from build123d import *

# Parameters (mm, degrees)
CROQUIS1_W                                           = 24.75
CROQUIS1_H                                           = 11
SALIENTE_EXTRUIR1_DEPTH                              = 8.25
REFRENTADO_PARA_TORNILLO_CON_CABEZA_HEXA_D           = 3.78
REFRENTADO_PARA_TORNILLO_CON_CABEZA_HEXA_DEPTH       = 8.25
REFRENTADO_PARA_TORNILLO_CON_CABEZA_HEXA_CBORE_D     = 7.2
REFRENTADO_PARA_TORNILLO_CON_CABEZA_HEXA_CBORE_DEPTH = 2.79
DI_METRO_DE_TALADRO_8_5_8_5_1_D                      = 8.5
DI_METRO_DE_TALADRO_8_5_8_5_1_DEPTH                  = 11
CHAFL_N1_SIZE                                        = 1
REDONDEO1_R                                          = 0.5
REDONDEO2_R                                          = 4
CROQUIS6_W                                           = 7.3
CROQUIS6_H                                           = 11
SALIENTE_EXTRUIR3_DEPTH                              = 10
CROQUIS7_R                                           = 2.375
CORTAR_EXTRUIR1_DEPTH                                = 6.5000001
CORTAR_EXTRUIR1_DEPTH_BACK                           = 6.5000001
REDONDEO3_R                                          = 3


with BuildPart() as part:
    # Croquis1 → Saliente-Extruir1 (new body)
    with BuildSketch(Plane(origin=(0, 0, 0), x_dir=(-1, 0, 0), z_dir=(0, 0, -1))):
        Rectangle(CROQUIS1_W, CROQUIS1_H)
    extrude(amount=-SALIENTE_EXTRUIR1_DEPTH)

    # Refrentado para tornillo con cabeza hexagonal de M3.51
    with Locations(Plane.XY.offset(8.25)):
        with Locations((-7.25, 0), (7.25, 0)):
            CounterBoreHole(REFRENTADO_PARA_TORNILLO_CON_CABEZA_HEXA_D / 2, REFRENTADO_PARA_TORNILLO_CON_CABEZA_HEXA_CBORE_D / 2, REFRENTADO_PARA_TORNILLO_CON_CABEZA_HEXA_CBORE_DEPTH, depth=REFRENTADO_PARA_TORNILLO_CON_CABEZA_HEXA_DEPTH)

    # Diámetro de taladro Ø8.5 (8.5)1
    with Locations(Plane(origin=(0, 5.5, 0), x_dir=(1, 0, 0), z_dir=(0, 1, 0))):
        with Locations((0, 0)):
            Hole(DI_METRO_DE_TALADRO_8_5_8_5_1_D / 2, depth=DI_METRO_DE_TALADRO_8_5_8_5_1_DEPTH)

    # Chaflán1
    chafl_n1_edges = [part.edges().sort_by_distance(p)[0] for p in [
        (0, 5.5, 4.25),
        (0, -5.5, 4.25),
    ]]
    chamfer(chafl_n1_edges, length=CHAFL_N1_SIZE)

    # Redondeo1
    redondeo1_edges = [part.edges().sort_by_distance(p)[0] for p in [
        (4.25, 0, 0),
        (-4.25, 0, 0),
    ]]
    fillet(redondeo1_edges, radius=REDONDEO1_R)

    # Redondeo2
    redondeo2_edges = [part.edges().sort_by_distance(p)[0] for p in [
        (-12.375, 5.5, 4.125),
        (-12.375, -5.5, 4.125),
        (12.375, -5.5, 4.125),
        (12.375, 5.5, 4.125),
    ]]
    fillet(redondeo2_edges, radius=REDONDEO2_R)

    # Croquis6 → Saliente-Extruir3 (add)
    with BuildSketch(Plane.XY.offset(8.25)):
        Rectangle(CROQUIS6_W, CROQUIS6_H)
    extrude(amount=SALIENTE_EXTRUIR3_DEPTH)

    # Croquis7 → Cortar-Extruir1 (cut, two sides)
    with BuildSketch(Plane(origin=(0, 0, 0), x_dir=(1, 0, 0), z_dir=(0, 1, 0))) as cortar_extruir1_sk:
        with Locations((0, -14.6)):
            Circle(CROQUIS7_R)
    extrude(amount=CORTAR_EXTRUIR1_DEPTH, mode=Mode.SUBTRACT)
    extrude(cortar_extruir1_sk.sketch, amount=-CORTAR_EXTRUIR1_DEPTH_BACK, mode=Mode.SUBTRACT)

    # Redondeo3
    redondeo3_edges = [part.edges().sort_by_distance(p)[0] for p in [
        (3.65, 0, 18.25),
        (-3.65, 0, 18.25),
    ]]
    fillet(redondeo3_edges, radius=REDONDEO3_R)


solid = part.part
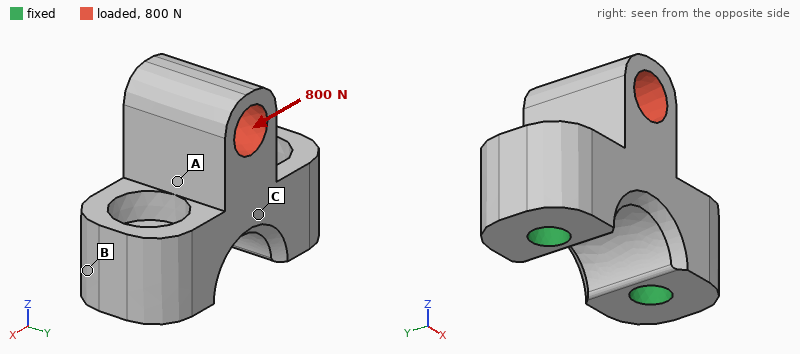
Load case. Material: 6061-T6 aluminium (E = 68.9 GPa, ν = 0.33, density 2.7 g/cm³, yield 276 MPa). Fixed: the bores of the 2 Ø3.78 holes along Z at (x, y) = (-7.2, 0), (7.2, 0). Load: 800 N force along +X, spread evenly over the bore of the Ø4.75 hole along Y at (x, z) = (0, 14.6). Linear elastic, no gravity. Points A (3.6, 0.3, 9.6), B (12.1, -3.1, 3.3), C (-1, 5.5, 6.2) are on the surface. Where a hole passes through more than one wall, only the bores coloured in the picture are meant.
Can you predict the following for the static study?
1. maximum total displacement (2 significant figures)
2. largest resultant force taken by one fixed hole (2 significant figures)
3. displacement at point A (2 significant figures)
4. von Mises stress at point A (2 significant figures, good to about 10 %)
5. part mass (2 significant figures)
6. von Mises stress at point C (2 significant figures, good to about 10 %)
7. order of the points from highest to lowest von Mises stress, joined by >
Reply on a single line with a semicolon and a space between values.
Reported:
31 µm; 860 N; 7.2 µm; 43 MPa; 5.5 g; 16 MPa; A > C > B
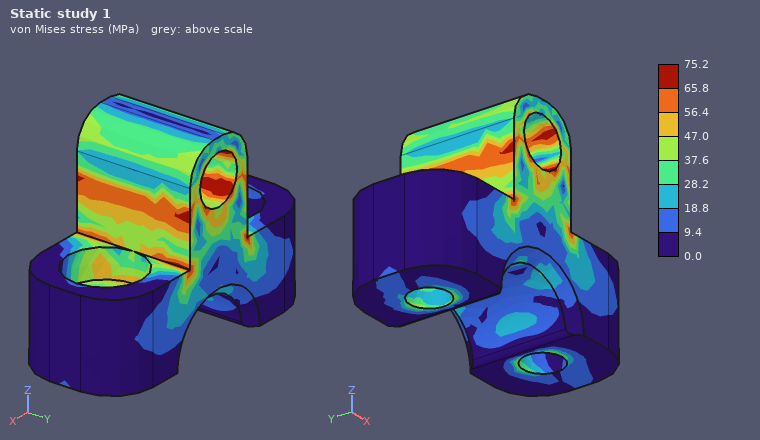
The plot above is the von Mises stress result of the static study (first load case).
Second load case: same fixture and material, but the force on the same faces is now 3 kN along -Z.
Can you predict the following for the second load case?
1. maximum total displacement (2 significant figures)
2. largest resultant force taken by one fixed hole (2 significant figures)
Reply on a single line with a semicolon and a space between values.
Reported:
21 µm; 1.7 kN
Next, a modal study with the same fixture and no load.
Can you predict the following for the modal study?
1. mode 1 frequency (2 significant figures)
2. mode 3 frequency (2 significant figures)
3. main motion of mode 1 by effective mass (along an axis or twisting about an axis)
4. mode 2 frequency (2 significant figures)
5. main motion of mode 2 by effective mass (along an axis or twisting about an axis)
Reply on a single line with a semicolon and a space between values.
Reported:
24 kHz; 58 kHz; along Y; 30 kHz; along X
